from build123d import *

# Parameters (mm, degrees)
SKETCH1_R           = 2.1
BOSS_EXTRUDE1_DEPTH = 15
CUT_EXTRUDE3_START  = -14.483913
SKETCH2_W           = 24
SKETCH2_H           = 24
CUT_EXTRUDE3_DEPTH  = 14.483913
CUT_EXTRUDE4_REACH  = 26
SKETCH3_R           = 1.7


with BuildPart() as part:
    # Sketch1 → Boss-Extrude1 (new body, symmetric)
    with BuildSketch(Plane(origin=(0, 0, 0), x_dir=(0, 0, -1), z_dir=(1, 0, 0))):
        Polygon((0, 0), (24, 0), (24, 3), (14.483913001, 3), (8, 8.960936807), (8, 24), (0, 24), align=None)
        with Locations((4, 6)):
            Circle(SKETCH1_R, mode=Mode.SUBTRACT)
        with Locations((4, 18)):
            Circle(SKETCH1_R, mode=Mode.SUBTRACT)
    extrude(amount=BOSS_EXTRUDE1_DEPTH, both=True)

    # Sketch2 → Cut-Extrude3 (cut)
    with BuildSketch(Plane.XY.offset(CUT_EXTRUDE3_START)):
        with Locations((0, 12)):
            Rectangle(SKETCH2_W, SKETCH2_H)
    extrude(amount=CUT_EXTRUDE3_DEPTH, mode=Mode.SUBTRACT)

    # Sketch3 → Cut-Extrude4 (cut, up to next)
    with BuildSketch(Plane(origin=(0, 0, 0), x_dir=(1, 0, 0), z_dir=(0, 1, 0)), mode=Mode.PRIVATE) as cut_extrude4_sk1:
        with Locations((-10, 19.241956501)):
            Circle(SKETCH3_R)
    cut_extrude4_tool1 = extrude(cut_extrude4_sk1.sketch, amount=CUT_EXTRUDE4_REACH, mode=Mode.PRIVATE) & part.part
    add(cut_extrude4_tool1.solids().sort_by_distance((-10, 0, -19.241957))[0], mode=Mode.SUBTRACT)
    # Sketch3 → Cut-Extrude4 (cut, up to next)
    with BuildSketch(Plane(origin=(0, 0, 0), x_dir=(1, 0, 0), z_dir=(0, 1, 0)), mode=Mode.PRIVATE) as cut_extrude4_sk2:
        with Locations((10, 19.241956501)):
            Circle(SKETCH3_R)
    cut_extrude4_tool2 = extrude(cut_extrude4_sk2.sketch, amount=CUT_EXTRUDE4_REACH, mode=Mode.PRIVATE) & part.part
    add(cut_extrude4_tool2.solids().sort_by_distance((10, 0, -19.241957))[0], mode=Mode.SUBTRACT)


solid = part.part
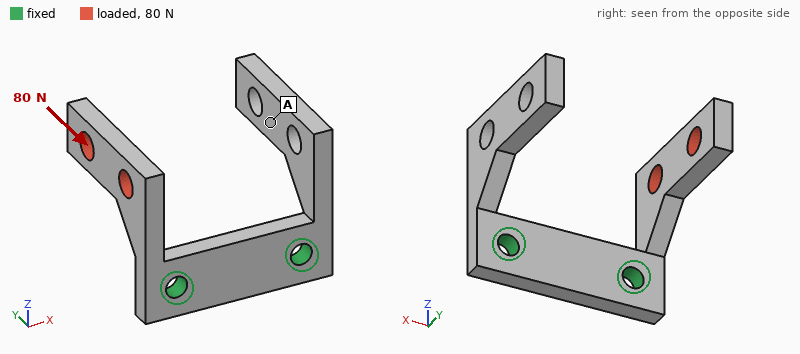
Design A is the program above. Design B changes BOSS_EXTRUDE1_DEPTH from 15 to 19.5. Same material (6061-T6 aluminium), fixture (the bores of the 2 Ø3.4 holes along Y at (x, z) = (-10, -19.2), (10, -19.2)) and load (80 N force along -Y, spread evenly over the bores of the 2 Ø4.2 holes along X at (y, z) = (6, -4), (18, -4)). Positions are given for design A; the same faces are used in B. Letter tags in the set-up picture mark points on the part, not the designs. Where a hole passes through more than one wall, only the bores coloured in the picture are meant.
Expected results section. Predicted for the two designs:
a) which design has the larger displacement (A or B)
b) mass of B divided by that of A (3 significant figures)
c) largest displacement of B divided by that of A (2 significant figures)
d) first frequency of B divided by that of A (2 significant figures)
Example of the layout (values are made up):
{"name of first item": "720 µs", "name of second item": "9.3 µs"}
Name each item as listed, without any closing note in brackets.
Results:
{"which design has the larger displacement": "A", "mass of B divided by that of A": "2.03", "largest displacement of B divided by that of A": "0.63", "first frequency of B divided by that of A": "0.88"}
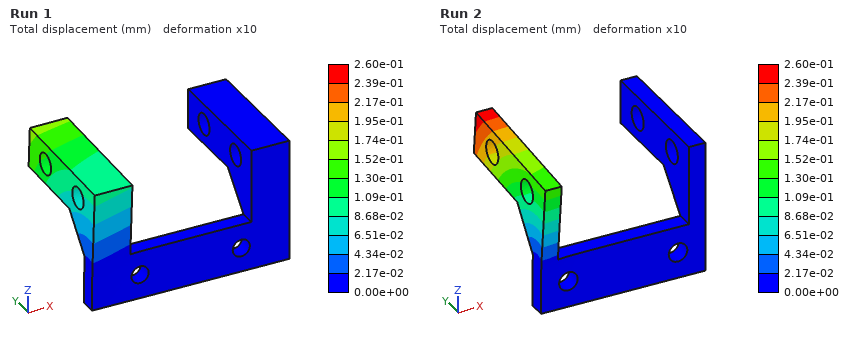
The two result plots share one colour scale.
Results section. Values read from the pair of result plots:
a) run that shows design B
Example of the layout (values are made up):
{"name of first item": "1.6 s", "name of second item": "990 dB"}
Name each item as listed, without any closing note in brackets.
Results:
{"run that shows design B": "Run 1"}
